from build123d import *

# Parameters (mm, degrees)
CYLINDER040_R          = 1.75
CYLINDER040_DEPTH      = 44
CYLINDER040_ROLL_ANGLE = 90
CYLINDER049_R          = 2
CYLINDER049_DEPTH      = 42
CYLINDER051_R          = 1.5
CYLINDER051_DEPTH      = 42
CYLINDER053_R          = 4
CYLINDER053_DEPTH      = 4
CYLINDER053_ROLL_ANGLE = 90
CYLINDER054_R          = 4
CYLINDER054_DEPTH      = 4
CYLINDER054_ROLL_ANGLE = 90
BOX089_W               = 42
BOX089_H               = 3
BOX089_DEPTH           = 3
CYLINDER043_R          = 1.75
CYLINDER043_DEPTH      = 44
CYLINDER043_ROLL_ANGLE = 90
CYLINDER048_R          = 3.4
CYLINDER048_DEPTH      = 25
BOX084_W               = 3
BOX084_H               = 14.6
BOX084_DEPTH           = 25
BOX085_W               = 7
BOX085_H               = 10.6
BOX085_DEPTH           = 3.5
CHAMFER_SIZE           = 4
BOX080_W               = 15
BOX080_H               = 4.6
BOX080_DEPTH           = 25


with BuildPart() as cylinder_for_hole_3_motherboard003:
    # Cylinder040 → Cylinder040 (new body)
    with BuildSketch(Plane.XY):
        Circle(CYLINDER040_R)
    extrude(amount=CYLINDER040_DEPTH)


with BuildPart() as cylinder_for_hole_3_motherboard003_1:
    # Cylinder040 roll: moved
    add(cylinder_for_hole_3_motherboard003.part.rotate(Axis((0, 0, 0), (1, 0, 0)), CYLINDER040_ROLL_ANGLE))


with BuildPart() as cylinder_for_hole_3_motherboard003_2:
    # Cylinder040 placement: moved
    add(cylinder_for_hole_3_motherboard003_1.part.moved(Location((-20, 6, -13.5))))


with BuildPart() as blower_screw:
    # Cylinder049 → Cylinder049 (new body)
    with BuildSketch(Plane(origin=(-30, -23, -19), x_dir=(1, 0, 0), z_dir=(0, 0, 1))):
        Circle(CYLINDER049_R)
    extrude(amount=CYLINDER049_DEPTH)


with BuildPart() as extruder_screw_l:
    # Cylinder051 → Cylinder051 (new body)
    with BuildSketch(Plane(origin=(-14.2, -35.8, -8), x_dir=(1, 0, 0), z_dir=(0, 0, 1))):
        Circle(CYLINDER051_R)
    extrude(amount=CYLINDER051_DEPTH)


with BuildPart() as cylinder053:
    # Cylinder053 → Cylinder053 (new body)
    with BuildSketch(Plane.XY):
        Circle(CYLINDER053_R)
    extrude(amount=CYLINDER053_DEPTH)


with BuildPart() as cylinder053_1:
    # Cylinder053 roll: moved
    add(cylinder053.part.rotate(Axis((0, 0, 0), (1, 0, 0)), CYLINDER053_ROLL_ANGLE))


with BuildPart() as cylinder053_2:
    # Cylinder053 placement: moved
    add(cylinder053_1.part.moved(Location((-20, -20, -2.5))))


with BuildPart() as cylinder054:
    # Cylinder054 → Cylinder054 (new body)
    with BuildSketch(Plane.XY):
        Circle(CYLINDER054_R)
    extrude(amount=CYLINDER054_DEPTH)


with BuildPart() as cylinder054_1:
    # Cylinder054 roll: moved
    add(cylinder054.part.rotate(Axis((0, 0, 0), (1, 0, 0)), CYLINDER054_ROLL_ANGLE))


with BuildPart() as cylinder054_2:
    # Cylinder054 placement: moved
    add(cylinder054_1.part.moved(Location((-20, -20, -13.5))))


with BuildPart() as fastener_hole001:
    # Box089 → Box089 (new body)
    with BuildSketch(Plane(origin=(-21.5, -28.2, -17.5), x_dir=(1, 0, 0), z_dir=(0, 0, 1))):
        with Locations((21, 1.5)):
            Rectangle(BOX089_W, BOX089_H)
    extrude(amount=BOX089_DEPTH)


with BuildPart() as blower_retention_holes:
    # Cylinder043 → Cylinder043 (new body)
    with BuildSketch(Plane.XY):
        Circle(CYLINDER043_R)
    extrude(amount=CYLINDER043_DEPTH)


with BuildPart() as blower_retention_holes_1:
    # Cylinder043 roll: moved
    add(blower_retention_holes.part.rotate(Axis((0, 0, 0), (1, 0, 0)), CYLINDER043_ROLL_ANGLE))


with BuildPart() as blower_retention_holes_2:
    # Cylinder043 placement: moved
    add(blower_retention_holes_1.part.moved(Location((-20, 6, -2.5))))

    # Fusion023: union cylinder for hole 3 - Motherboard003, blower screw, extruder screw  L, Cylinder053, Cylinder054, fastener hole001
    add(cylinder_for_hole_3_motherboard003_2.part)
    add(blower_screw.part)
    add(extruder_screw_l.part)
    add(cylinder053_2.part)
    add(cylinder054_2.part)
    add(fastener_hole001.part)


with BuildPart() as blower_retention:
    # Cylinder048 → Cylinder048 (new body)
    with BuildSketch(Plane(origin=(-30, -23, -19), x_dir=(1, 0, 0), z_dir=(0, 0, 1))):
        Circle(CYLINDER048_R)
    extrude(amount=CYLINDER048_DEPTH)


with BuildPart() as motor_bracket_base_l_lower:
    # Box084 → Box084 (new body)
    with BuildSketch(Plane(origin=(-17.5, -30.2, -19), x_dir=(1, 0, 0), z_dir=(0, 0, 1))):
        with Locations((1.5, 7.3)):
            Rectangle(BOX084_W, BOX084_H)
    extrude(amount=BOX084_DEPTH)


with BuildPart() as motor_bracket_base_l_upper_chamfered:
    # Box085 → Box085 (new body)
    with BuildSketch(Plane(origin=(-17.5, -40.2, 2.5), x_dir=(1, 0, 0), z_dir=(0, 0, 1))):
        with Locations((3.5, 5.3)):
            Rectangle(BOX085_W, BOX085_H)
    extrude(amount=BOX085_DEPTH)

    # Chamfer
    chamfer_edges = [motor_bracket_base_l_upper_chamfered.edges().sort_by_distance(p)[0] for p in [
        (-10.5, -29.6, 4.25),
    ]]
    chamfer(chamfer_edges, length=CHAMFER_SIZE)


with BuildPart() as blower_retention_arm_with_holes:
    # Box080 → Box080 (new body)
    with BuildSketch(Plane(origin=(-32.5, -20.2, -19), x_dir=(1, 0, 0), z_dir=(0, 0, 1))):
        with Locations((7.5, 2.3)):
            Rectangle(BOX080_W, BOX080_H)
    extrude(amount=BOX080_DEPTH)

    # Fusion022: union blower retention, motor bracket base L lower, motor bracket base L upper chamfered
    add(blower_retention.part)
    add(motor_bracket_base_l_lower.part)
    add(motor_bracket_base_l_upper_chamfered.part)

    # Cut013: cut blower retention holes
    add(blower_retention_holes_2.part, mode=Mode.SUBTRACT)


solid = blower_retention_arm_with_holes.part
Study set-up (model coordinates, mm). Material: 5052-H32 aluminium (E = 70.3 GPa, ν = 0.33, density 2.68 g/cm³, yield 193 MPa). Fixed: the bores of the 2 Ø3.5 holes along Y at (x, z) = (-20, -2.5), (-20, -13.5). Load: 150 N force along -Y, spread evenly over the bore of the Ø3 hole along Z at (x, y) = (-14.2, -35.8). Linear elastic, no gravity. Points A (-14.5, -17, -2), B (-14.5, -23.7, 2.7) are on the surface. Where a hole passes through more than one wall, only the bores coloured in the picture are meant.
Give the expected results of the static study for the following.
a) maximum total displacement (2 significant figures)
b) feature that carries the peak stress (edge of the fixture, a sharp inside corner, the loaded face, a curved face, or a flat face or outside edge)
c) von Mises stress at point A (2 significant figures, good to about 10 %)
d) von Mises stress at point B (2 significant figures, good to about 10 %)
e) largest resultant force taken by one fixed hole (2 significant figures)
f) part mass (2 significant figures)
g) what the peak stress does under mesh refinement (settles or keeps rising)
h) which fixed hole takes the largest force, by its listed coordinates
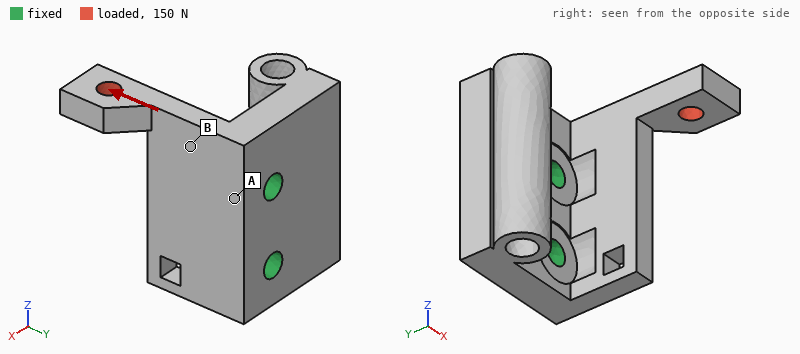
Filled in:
53 µm
a sharp inside corner
5.6 MPa
23 MPa
200 N
9.1 g
keeps rising
(-20, -2.5)
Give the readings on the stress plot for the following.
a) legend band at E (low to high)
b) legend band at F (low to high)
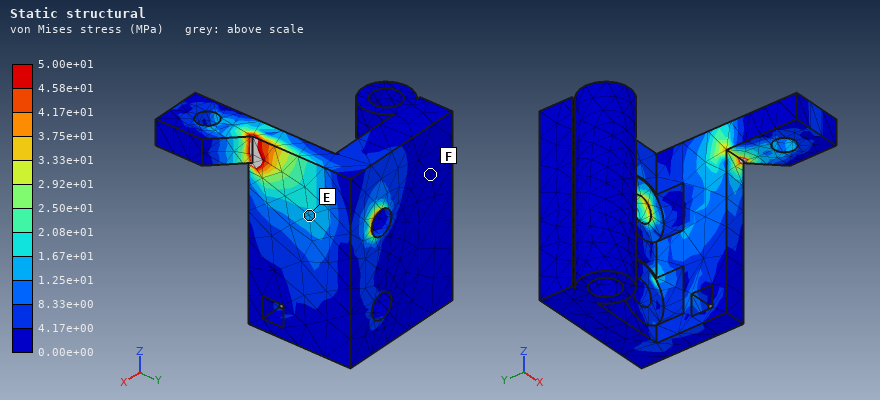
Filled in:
1.25e+01 to 1.67e+01 MPa
0.00e+00 to 4.17e+00 MPa
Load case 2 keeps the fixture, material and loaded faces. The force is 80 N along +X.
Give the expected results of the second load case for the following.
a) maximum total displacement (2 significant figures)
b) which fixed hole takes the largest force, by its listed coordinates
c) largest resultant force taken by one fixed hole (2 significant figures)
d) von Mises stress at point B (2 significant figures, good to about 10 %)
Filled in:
0.15 mm
(-20, -2.5)
110 N
55 MPa
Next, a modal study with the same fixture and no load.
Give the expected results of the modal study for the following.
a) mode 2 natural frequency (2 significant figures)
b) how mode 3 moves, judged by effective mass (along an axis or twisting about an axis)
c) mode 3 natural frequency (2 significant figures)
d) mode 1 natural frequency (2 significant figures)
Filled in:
12 kHz
along Y
14 kHz
5600 Hz
